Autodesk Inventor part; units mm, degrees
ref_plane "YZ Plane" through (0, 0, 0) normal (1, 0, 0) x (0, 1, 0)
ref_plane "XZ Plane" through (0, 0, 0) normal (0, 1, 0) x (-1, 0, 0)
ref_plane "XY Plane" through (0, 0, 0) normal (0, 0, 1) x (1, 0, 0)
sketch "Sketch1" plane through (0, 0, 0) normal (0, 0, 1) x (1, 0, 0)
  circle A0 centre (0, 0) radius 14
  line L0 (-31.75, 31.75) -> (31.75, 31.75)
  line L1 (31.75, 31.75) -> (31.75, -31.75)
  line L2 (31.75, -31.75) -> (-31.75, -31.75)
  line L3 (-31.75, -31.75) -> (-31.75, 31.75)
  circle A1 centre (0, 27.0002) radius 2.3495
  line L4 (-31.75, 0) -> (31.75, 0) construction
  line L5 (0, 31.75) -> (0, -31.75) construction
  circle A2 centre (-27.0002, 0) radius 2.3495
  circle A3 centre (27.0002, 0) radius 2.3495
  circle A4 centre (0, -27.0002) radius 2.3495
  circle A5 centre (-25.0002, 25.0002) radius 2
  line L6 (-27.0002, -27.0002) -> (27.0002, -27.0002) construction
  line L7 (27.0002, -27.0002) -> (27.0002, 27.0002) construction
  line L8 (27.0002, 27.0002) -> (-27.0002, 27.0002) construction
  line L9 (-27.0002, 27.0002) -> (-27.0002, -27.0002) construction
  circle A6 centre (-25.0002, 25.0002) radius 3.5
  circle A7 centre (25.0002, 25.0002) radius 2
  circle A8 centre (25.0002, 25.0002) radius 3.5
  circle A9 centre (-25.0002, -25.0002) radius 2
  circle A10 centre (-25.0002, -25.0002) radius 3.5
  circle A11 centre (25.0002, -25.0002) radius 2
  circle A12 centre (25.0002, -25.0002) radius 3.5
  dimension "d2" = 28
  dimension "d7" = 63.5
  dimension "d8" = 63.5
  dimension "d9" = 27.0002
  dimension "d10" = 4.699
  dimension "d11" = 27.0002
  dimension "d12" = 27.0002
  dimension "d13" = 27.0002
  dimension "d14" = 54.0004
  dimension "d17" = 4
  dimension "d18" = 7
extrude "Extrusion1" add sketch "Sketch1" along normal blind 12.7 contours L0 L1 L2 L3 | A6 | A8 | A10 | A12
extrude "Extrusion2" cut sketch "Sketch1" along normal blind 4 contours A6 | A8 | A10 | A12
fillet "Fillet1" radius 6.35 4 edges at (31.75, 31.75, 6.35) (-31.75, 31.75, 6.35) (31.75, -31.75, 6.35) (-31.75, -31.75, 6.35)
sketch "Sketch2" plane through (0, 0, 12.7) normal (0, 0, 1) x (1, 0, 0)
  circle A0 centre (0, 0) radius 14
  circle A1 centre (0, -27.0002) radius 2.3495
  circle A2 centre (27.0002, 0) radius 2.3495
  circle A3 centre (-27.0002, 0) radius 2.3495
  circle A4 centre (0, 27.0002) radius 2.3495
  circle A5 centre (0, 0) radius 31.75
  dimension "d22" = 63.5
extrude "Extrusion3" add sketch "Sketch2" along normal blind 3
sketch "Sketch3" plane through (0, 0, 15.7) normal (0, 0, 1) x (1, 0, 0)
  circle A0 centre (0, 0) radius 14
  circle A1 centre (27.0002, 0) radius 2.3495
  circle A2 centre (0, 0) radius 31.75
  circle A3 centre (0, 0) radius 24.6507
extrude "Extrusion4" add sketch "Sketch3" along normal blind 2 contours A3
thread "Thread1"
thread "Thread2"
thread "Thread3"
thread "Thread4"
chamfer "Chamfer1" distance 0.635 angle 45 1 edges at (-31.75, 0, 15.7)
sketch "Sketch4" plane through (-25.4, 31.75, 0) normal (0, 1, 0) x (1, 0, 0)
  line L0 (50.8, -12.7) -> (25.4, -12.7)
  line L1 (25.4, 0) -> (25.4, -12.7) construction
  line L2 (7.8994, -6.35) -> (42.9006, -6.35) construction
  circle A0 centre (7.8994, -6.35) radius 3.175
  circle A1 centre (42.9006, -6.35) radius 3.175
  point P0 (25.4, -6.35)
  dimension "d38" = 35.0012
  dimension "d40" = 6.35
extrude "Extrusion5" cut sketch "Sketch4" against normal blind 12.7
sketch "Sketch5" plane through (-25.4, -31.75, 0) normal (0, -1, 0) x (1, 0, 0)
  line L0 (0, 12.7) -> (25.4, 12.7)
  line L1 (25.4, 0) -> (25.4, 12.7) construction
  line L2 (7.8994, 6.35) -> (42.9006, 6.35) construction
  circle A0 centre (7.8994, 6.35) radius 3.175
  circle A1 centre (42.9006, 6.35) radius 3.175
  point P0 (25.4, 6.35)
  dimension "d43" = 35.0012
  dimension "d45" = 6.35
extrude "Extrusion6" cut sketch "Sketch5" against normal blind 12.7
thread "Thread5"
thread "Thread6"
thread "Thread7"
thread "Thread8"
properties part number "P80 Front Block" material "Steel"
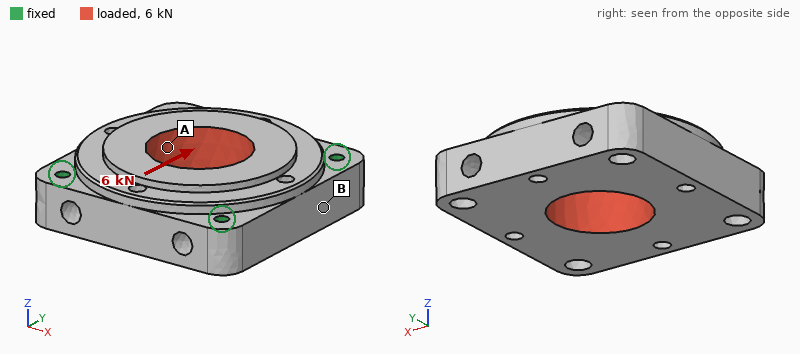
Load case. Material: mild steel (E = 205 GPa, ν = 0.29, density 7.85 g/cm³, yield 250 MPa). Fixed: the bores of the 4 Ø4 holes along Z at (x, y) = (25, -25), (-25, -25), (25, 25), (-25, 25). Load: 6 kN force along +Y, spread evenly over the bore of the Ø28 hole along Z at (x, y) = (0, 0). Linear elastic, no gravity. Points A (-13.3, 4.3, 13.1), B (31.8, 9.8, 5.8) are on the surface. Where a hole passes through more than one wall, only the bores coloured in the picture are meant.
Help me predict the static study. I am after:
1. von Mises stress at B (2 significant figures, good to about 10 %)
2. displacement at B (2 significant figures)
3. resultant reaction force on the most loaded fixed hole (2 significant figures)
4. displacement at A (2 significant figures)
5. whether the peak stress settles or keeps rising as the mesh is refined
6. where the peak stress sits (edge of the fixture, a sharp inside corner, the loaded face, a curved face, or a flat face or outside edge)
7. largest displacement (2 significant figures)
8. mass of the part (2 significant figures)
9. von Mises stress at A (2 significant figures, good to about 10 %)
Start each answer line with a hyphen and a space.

- 3.5 MPa
- 0.44 µm
- 1.6 kN
- 1.1 µm
- keeps rising
- edge of the fixture
- 1.6 µm
- 390 g
- 8.2 MPa
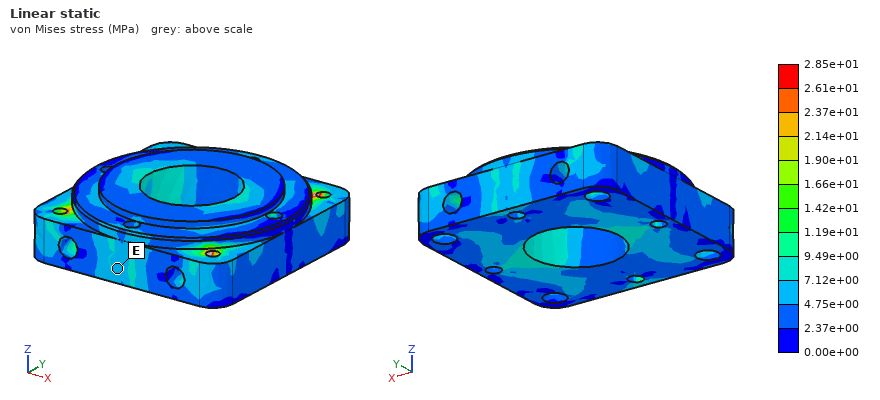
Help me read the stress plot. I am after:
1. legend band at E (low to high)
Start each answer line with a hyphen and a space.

- 4.75e+00 to 7.12e+00 MPa
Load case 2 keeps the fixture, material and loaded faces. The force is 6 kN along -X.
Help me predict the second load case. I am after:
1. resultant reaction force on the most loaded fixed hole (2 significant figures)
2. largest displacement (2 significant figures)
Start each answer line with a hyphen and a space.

- 1.6 kN
- 1.7 µm
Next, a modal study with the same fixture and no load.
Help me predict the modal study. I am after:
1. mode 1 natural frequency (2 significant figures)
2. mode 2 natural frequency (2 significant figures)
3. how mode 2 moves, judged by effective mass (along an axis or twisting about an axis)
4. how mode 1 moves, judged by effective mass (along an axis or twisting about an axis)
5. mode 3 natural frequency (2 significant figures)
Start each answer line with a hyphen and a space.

- 12 kHz
- 16 kHz
- twisting about X
- along Z
- 17 kHz
